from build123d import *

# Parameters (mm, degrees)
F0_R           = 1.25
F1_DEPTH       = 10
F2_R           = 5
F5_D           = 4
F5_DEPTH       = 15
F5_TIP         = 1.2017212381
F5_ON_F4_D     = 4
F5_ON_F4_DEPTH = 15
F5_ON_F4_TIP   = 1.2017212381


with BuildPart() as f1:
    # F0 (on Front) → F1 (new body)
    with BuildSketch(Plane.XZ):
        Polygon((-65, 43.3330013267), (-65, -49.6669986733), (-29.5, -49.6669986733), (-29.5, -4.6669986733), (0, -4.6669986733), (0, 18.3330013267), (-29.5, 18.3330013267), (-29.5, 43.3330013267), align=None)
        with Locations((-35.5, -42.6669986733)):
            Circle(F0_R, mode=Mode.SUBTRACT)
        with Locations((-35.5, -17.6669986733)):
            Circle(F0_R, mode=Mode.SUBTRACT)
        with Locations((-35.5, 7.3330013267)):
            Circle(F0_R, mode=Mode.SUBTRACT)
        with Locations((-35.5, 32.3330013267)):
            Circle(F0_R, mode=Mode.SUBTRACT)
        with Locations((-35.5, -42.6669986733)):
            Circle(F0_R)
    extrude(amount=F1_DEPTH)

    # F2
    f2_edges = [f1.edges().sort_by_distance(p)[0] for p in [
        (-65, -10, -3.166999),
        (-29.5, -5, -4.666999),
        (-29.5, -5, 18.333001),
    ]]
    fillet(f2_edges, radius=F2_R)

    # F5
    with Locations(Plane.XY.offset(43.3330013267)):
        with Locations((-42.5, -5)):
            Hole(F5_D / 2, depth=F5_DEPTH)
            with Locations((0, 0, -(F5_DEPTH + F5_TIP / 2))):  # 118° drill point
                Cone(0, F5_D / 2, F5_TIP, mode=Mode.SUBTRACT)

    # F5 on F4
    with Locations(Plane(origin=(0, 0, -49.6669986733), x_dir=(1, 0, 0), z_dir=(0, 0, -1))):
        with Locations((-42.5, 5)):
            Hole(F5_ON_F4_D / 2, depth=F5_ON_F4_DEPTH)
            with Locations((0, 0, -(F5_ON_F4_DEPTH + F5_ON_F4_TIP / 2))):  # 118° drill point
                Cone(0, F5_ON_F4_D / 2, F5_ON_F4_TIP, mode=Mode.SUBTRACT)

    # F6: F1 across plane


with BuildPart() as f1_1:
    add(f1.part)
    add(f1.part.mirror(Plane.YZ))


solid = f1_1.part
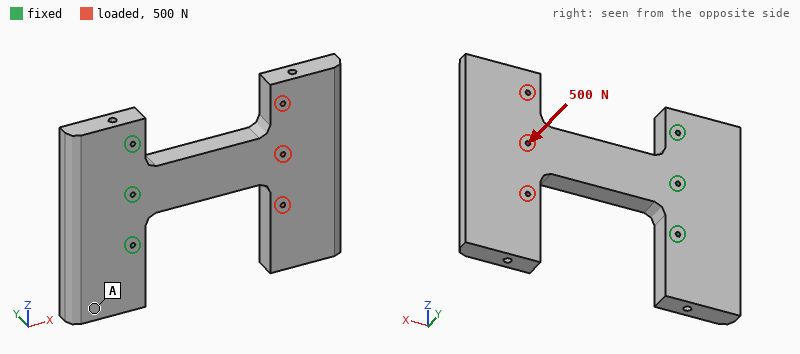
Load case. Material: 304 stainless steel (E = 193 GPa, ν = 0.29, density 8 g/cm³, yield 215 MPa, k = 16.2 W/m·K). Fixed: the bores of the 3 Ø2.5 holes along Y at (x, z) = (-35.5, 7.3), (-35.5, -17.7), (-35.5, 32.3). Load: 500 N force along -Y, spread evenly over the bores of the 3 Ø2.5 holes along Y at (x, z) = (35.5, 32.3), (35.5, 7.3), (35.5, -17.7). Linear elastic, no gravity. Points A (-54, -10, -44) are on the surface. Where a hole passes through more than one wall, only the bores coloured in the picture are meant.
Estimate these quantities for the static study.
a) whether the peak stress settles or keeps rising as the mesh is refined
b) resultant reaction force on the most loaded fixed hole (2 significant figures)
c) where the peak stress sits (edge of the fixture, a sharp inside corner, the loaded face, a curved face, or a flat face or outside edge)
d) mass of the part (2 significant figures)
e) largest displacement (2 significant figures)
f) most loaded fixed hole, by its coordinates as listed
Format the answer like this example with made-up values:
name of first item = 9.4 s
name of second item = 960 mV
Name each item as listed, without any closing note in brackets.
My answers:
whether the peak stress settles or keeps rising as the mesh is refined = keeps rising
resultant reaction force on the most loaded fixed hole = 800 N
where the peak stress sits = edge of the fixture
mass of the part = 620 g
largest displacement = 0.28 mm
most loaded fixed hole, by its coordinates as listed = (-35.5, 7.3)
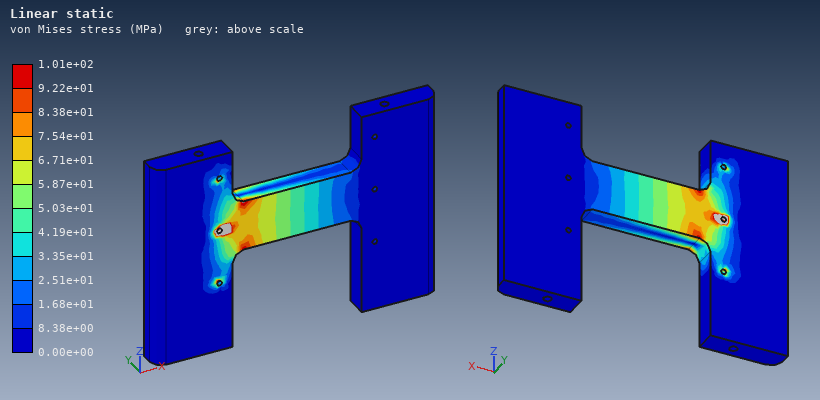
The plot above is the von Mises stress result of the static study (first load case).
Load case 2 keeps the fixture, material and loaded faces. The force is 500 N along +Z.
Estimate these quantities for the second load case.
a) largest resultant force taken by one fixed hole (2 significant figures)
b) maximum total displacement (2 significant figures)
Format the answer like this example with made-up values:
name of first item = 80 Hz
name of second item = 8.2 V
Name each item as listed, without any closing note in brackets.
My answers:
largest resultant force taken by one fixed hole = 780 N
maximum total displacement = 62 µm
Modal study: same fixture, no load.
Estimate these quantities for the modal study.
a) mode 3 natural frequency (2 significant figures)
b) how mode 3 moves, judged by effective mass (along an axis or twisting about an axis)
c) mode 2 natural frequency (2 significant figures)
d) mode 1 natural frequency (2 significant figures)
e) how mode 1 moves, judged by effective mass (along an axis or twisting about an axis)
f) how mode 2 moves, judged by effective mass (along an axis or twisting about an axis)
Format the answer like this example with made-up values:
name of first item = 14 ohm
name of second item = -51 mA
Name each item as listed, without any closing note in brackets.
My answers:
mode 3 natural frequency = 910 Hz
how mode 3 moves, judged by effective mass = twisting about X
mode 2 natural frequency = 860 Hz
mode 1 natural frequency = 410 Hz
how mode 1 moves, judged by effective mass = along Y
how mode 2 moves, judged by effective mass = along Z
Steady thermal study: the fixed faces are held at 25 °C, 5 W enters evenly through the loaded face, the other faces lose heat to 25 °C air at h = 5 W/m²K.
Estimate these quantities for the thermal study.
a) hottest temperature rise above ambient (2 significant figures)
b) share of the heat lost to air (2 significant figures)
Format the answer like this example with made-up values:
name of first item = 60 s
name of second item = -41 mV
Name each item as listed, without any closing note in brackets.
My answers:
hottest temperature rise above ambient = 55 K
share of the heat lost to air = 53 %
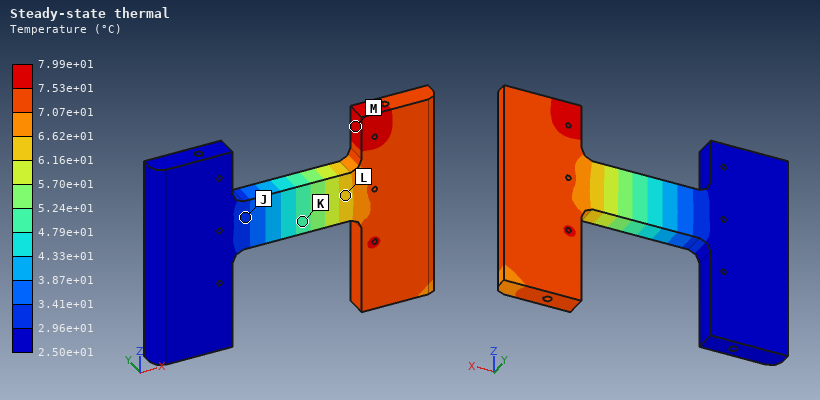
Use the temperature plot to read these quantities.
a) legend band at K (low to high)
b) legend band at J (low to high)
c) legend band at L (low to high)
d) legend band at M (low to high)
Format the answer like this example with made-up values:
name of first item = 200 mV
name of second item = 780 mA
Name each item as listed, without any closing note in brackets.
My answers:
legend band at K = 4.79e+01 to 5.24e+01 °C
legend band at J = 2.96e+01 to 3.41e+01 °C
legend band at L = 6.16e+01 to 6.62e+01 °C
legend band at M = 7.53e+01 to 7.99e+01 °C
